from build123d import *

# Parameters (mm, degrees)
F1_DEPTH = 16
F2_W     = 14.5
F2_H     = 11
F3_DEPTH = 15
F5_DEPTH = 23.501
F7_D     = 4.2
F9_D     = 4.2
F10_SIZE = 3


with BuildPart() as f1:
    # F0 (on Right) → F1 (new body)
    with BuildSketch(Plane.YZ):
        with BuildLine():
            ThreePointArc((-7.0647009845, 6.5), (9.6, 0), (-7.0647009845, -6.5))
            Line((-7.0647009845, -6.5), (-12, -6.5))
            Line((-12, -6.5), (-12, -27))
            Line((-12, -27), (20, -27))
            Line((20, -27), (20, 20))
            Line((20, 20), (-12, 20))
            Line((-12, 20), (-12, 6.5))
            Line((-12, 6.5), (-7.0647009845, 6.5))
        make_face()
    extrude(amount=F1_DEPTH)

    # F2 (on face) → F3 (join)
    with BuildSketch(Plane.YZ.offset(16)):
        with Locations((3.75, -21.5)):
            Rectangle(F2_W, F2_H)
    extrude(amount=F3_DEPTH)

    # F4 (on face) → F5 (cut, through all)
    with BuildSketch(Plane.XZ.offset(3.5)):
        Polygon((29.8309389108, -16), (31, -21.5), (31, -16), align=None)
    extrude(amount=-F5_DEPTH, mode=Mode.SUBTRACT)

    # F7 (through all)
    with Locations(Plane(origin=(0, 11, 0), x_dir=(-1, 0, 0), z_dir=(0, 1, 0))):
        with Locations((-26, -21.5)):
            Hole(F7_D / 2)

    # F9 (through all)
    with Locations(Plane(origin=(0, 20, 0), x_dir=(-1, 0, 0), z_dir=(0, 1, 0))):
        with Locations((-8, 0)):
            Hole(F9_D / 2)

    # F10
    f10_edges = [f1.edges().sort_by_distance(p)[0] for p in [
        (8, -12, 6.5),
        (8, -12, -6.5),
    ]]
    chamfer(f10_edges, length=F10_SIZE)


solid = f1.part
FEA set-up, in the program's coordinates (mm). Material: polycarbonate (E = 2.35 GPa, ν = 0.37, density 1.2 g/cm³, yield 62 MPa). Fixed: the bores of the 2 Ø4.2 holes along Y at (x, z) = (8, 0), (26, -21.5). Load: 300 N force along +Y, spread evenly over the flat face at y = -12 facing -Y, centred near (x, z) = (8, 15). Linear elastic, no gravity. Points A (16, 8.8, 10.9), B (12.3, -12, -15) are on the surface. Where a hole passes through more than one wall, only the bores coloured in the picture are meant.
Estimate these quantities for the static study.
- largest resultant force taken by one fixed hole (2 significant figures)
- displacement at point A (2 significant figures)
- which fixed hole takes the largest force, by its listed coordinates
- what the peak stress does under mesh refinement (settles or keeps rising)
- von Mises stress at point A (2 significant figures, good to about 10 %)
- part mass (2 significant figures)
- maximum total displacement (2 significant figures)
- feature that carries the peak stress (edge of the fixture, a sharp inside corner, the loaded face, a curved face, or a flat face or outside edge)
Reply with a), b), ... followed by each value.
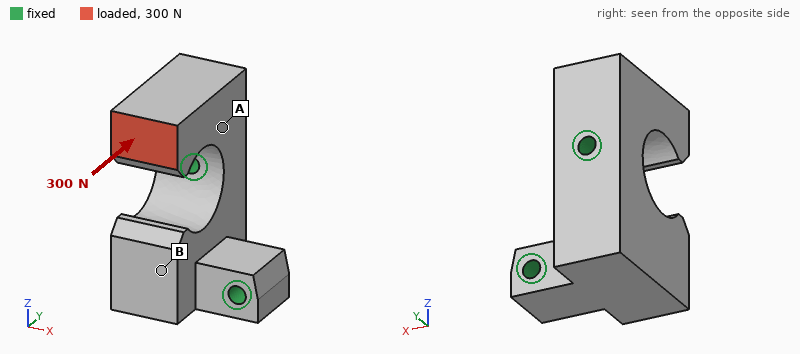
a) 320 N
b) 0.090 mm
c) (8, 0)
d) keeps rising
e) 3.1 MPa
f) 25 g
g) 0.29 mm
h) edge of the fixture
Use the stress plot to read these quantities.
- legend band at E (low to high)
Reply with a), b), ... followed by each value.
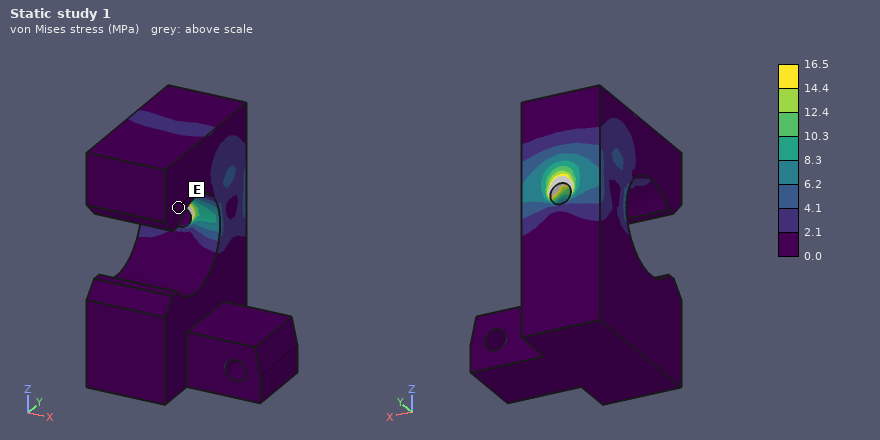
a) 0.0 to 2.1 MPa
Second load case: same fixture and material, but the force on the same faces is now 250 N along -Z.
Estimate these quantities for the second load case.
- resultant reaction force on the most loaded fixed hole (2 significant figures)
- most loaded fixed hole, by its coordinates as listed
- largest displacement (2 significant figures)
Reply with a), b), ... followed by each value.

a) 250 N
b) (8, 0)
c) 0.75 mm
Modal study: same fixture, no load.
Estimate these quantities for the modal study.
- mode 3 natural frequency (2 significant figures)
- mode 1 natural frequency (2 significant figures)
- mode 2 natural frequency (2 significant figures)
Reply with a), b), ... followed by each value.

a) 2800 Hz
b) 1900 Hz
c) 2000 Hz
